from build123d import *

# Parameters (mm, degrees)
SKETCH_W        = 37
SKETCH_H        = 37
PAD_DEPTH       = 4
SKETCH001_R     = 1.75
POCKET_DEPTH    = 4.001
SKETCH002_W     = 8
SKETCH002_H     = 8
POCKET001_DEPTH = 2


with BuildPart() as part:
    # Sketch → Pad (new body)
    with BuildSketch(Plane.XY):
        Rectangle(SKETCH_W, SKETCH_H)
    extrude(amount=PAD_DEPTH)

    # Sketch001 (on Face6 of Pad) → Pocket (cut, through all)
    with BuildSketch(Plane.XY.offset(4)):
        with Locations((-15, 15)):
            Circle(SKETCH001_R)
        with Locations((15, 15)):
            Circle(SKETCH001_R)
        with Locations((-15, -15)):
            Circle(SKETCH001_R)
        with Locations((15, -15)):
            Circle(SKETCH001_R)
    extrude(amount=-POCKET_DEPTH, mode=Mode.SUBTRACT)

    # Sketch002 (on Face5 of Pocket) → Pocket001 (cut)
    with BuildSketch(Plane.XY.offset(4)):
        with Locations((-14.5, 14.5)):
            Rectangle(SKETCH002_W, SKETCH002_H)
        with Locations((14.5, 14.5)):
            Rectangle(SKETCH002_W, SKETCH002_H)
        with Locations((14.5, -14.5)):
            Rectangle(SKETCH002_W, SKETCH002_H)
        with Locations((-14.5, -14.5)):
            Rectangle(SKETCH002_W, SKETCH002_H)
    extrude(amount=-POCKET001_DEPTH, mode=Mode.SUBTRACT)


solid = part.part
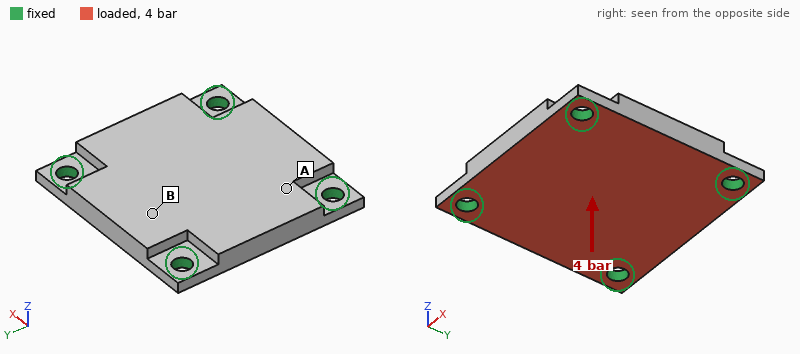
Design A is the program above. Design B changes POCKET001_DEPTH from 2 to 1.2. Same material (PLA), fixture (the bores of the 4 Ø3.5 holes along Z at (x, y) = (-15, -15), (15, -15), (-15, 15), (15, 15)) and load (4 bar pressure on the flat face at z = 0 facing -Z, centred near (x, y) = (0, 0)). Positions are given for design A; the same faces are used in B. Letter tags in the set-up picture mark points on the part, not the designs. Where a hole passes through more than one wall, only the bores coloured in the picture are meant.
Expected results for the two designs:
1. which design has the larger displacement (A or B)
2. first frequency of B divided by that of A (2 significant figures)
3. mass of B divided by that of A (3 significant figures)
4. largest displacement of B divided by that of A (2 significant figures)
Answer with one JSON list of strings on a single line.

["A", "1.1", "1.04", "0.85"]
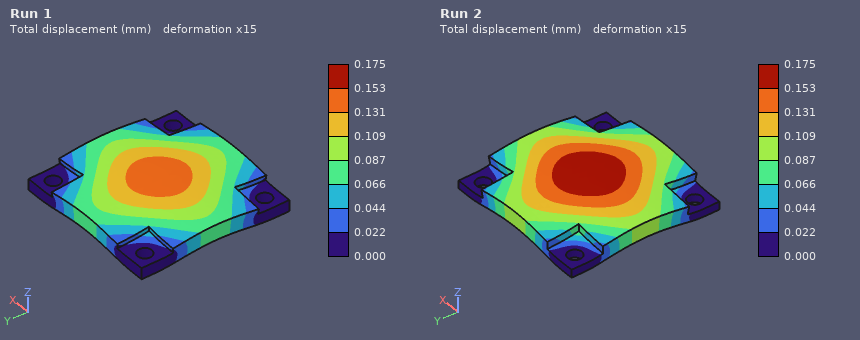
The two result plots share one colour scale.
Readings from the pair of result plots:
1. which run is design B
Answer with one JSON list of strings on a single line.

["Run 1"]
